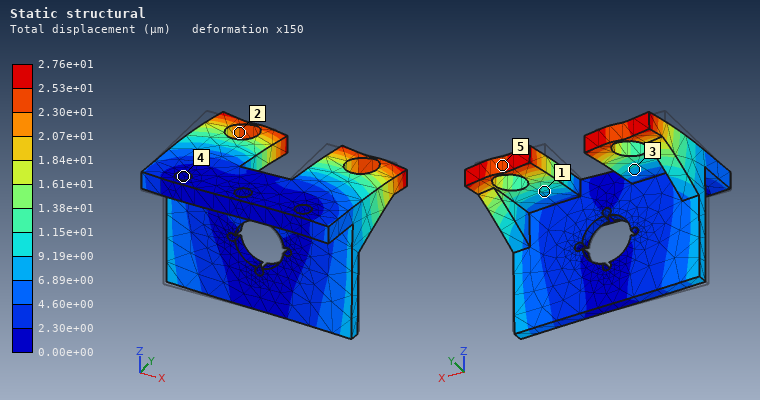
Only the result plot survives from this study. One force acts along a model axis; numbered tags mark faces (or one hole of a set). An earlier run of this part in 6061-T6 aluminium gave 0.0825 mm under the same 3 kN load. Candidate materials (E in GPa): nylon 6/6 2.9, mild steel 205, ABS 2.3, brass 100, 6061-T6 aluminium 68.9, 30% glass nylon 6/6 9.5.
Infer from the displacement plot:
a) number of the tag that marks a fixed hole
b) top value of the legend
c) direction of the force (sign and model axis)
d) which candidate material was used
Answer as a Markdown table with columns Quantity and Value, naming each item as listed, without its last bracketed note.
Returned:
| Quantity | Value |
|---|---|
| number of the tag that marks a fixed hole | 4 |
| top value of the legend | 2.76e+01 µm |
| direction of the force | +X |
| which candidate material was used | mild steel |
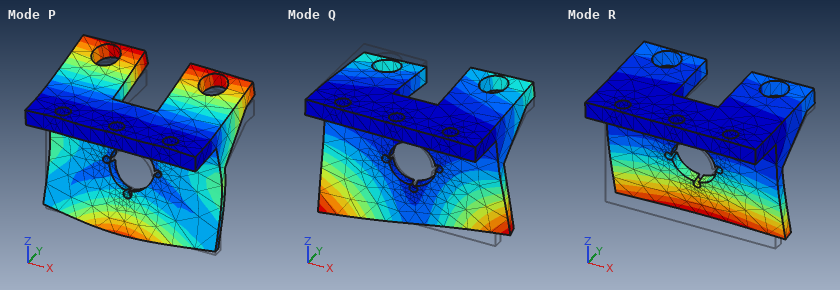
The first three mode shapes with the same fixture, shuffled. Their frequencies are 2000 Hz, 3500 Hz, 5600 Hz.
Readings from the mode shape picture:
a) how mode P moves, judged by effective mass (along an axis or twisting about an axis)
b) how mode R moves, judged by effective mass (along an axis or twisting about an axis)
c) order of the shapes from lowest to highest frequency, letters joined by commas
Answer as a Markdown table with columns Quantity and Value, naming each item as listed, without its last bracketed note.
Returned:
| Quantity | Value |
|---|---|
| how mode P moves, judged by effective mass | along Z |
| how mode R moves, judged by effective mass | along Y |
| order of the shapes from lowest to highest frequency, letters joined by commas | R, Q, P |
